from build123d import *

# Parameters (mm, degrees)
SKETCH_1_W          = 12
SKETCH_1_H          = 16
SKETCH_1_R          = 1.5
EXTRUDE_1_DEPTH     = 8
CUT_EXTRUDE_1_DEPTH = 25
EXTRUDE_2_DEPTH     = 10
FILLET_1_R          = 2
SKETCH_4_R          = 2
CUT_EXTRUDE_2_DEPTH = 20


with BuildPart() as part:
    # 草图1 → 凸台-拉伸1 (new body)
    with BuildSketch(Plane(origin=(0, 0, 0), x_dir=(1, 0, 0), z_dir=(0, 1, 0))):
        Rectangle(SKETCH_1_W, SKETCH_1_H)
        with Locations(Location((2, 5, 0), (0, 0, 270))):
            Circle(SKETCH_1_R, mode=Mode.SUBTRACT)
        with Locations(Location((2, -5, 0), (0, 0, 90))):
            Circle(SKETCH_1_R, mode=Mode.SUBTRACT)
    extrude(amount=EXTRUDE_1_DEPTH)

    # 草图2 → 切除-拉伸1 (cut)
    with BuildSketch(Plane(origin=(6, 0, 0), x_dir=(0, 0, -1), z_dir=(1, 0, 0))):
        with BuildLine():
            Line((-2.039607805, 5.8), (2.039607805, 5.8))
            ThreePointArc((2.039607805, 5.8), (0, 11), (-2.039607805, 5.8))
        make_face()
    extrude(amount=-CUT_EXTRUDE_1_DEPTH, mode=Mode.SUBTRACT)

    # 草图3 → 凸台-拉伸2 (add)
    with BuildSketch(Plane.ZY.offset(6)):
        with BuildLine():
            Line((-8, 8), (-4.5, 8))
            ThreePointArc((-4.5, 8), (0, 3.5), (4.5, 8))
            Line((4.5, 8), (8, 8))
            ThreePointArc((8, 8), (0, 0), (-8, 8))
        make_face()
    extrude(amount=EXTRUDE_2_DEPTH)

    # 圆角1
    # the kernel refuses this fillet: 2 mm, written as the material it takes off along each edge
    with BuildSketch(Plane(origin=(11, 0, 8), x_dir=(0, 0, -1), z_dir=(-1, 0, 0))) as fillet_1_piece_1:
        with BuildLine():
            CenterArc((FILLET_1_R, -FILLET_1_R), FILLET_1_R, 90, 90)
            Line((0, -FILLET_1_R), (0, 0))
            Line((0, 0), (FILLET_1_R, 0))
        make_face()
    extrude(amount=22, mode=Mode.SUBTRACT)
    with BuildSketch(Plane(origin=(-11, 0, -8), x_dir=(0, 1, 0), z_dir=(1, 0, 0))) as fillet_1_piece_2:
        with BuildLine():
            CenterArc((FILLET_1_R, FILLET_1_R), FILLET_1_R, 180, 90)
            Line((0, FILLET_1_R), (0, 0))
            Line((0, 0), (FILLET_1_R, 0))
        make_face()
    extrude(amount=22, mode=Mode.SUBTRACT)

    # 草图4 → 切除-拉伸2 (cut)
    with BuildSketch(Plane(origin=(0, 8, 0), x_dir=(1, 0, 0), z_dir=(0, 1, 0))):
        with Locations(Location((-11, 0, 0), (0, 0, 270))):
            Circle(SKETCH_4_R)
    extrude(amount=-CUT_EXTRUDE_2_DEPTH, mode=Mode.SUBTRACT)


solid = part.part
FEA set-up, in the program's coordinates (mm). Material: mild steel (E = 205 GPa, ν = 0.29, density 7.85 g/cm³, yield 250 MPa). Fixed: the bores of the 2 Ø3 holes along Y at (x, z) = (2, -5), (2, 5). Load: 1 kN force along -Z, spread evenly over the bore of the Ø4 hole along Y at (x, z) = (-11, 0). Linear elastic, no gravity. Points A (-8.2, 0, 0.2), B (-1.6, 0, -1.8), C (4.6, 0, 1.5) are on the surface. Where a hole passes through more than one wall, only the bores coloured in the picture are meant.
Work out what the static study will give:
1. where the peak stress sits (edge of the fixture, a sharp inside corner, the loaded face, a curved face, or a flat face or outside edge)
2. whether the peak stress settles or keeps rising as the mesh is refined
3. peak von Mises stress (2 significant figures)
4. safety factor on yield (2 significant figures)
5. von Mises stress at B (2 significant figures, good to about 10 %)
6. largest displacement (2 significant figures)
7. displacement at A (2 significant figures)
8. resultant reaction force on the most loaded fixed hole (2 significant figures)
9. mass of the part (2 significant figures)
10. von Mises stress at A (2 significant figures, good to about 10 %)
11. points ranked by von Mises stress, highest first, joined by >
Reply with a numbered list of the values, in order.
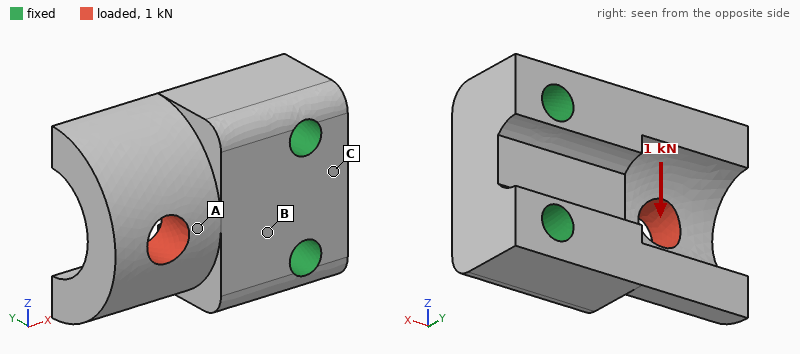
1. the loaded face
2. settles
3. 110 MPa
4. 2.3
5. 27 MPa
6. 6.7 µm
7. 2.8 µm
8. 1.2 kN
9. 15 g
10. 50 MPa
11. A > B > C
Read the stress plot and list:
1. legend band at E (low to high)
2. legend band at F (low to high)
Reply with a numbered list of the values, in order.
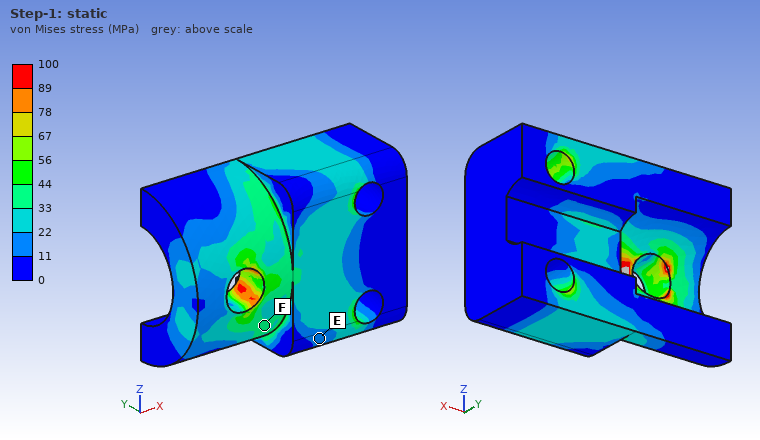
1. 11 to 22 MPa
2. 33 to 44 MPa
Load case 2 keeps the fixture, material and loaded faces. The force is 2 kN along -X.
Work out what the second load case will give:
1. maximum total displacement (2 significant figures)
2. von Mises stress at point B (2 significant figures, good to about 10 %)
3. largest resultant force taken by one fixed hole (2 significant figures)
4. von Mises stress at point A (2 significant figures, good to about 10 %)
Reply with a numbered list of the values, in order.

1. 9.1 µm
2. 44 MPa
3. 1.0 kN
4. 50 MPa
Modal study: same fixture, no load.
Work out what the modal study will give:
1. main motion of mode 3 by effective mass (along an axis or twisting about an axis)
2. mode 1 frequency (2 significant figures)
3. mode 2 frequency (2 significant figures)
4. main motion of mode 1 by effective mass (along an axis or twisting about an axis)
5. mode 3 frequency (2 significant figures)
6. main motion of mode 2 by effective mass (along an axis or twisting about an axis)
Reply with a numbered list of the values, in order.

1. along Z
2. 22 kHz
3. 25 kHz
4. along Y
5. 38 kHz
6. along Z
